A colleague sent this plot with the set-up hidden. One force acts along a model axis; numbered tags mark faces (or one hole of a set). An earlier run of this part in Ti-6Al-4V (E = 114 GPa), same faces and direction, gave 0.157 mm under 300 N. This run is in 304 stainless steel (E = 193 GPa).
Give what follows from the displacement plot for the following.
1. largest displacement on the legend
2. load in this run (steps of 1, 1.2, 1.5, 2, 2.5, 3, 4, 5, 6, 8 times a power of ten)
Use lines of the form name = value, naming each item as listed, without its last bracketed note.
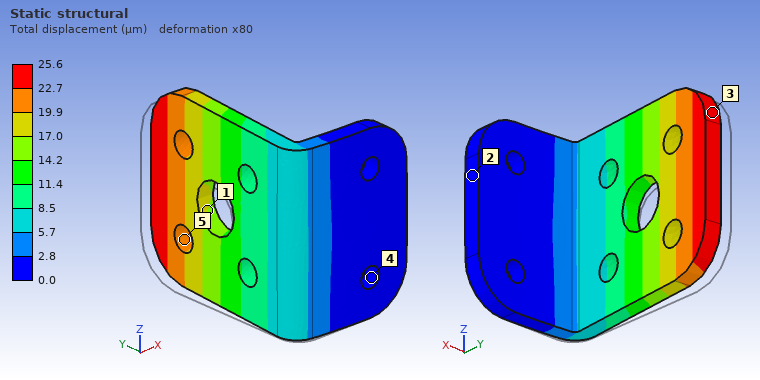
largest displacement on the legend = 25.6 µm
load in this run = 80 N
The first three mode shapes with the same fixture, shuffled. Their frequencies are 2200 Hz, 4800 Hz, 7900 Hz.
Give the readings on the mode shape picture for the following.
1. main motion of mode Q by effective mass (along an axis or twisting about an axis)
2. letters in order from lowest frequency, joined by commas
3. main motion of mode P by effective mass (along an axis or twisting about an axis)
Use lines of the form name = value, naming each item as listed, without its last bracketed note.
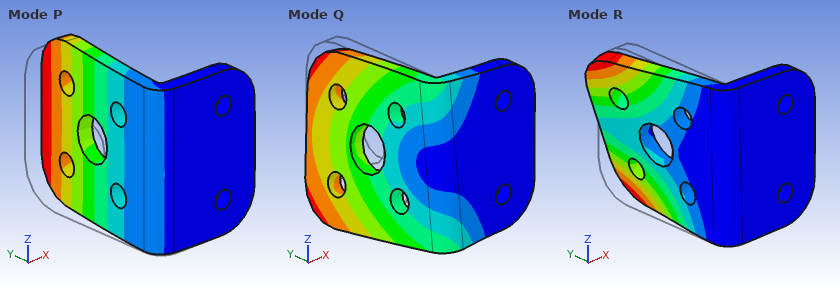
main motion of mode Q by effective mass = along Z
letters in order from lowest frequency, joined by commas = P, Q, R
main motion of mode P by effective mass = along X
